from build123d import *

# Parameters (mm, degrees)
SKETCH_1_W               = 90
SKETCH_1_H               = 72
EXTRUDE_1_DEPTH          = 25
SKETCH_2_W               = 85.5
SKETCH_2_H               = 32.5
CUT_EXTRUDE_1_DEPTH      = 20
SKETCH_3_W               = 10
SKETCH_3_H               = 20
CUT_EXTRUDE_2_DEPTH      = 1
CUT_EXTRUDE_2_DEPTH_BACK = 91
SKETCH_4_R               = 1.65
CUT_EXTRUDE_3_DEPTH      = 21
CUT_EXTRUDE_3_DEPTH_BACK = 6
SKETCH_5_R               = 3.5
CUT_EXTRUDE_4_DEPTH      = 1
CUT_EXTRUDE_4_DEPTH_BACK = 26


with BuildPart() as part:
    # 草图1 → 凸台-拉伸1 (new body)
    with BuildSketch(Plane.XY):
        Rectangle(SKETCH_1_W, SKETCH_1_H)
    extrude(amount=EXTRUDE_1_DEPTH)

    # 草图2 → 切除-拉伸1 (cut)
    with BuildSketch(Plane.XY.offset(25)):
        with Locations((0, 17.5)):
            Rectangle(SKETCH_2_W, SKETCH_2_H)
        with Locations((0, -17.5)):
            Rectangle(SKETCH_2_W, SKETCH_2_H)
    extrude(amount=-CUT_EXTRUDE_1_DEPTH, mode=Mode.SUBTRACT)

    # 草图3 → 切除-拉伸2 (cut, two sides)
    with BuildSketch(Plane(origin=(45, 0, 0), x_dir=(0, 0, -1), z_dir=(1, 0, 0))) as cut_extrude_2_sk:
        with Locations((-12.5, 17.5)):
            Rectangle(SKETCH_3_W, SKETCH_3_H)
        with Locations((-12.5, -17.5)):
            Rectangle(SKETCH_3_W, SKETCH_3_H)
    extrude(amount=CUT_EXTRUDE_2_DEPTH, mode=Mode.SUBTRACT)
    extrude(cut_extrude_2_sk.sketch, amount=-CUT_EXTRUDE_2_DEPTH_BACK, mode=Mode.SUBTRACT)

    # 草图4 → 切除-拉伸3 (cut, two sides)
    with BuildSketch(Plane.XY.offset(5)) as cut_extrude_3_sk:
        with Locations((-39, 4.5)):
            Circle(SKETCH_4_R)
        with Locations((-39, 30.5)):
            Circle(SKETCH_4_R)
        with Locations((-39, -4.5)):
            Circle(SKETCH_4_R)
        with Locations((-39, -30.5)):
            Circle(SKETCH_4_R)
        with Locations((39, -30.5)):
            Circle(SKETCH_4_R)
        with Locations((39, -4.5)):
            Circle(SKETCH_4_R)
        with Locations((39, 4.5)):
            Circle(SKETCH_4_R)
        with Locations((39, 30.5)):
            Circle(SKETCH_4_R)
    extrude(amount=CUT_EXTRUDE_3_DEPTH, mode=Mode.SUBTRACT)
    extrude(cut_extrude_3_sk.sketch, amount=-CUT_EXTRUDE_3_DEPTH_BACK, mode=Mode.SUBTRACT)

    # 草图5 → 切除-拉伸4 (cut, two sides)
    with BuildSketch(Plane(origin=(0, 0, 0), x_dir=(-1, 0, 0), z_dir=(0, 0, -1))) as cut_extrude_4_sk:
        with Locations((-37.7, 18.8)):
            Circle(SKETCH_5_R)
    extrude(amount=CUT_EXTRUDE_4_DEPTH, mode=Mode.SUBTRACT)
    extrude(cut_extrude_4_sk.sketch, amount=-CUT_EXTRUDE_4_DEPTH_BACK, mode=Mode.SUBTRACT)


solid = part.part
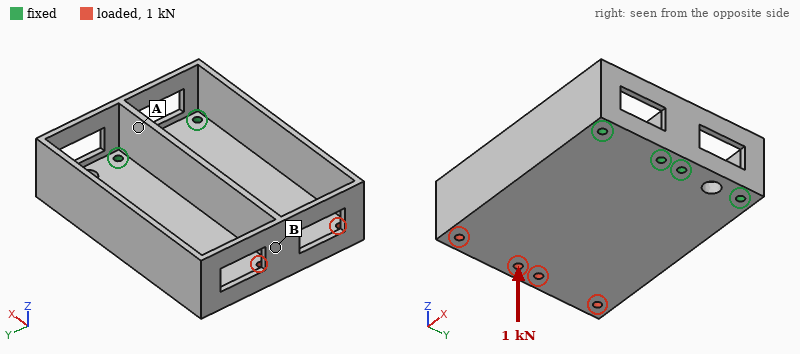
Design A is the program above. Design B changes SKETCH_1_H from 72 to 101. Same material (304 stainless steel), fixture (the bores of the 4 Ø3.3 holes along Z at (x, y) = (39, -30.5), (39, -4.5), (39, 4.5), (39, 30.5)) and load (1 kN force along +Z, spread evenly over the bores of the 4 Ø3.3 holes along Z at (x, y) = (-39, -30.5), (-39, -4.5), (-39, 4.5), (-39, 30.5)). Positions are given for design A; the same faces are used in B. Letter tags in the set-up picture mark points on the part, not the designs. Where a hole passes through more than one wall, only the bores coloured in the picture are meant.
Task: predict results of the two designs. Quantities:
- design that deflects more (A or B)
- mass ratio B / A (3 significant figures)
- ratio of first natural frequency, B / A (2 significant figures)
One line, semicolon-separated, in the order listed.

A; 2.34; 0.70
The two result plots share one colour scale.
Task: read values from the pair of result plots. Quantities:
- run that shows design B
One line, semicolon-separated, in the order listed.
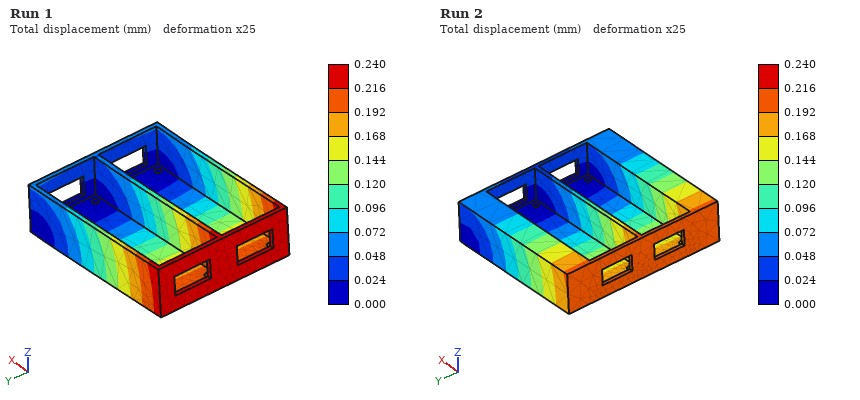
Run 2
